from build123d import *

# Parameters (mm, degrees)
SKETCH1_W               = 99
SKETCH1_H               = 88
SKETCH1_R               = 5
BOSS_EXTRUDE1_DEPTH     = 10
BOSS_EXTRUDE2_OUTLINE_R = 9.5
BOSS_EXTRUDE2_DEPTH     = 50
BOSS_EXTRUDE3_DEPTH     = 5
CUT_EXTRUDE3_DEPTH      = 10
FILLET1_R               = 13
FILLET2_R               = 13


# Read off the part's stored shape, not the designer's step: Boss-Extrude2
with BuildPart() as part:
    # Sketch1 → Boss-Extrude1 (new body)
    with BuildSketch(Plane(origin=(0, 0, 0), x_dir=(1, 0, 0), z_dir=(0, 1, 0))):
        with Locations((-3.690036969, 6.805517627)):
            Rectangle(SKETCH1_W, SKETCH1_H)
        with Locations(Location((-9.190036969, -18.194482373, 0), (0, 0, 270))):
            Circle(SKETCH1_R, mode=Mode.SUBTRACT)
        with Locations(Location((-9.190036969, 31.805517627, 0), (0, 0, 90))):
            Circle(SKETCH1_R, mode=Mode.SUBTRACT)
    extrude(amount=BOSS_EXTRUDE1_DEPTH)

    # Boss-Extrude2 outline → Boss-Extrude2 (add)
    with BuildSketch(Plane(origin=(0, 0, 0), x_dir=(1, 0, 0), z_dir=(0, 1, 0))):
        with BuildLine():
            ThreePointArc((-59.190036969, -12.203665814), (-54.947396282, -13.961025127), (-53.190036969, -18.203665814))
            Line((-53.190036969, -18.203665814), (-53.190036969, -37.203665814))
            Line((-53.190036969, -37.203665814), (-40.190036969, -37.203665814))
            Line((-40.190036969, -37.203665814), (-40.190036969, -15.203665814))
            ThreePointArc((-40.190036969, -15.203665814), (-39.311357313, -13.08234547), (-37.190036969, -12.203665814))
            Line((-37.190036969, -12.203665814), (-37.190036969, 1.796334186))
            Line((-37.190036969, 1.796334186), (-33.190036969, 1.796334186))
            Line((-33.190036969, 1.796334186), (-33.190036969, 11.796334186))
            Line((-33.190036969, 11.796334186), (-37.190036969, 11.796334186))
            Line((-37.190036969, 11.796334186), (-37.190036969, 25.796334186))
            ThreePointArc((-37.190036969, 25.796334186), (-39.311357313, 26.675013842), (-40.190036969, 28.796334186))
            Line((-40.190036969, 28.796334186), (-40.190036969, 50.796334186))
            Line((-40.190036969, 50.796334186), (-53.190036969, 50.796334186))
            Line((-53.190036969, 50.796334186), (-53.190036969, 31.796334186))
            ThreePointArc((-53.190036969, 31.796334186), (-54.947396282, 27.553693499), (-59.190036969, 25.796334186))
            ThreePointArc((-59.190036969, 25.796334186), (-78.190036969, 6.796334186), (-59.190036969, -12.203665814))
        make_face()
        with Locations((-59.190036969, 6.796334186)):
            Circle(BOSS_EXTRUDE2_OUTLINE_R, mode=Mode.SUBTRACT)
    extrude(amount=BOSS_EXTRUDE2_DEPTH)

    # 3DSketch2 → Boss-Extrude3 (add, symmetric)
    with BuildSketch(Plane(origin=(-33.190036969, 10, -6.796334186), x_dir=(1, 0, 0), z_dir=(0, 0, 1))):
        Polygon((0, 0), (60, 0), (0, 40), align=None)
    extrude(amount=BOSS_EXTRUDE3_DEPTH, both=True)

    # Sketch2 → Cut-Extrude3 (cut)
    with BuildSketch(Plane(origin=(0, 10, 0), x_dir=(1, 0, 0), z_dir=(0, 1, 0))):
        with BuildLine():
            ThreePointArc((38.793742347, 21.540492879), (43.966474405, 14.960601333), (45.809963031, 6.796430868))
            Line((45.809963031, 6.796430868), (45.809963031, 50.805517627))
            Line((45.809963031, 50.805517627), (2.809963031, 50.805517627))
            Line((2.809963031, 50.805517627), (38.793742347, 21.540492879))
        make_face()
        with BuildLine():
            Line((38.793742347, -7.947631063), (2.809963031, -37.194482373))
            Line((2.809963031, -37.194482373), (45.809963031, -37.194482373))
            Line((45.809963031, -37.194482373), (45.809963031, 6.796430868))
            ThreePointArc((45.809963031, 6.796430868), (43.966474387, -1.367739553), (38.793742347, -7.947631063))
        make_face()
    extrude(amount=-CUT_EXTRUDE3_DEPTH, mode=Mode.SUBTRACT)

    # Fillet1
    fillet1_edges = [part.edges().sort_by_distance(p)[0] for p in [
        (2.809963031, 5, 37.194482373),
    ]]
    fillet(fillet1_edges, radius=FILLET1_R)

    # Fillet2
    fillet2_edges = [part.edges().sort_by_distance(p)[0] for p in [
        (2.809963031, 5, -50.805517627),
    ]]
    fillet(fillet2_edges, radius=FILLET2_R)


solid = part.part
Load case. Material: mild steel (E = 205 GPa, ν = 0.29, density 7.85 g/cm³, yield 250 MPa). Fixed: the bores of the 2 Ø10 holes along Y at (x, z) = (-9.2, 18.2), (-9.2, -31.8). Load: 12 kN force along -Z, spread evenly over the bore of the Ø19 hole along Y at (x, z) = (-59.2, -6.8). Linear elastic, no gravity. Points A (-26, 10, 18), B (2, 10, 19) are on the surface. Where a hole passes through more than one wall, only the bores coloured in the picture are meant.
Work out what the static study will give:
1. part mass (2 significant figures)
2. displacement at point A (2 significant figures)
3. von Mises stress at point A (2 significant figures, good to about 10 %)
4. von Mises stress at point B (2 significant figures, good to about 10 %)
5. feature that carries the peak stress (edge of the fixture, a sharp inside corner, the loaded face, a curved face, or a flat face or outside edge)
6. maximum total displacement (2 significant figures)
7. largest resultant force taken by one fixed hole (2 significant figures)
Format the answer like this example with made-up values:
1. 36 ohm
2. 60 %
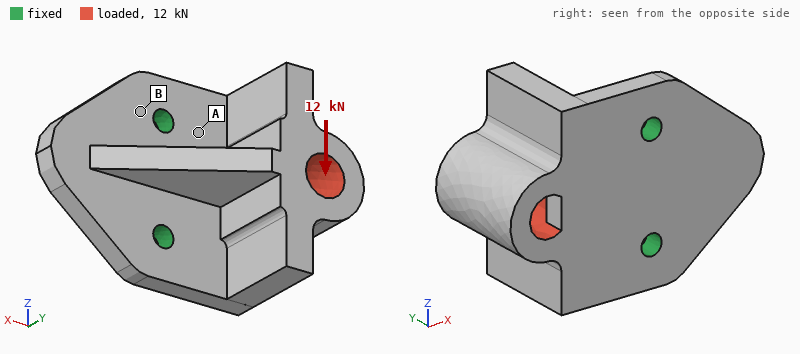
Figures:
1. 1.3 kg
2. 11 µm
3. 65 MPa
4. 16 MPa
5. a flat face or outside edge
6. 60 µm
7. 13 kN
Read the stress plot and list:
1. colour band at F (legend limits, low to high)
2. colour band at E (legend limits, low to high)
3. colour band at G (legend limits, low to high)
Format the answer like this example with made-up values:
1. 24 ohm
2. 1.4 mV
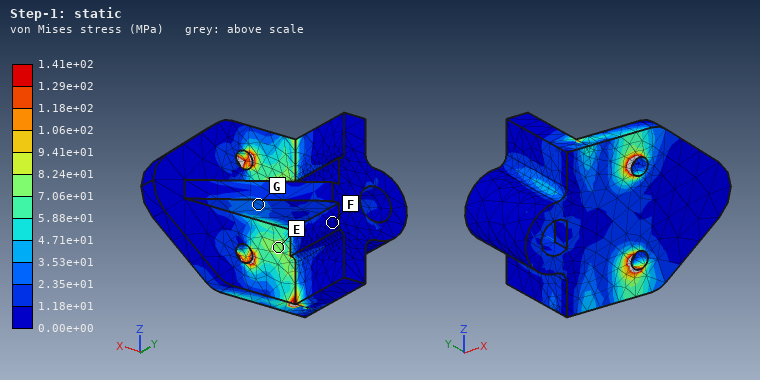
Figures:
1. 0.00e+00 to 1.18e+01 MPa
2. 7.06e+01 to 8.24e+01 MPa
3. 2.35e+01 to 3.53e+01 MPa
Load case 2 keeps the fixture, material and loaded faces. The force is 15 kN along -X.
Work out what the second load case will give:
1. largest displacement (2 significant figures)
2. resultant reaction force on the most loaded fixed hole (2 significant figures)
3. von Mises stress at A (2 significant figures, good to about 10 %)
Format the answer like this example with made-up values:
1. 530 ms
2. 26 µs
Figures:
1. 0.15 mm
2. 7.5 kN
3. 70 MPa
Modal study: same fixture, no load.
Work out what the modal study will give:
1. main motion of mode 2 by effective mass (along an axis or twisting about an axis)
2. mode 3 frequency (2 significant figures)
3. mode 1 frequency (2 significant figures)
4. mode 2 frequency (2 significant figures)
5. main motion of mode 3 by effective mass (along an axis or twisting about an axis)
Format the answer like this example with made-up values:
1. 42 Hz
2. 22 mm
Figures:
1. along Z
2. 5400 Hz
3. 1600 Hz
4. 2900 Hz
5. along Y
